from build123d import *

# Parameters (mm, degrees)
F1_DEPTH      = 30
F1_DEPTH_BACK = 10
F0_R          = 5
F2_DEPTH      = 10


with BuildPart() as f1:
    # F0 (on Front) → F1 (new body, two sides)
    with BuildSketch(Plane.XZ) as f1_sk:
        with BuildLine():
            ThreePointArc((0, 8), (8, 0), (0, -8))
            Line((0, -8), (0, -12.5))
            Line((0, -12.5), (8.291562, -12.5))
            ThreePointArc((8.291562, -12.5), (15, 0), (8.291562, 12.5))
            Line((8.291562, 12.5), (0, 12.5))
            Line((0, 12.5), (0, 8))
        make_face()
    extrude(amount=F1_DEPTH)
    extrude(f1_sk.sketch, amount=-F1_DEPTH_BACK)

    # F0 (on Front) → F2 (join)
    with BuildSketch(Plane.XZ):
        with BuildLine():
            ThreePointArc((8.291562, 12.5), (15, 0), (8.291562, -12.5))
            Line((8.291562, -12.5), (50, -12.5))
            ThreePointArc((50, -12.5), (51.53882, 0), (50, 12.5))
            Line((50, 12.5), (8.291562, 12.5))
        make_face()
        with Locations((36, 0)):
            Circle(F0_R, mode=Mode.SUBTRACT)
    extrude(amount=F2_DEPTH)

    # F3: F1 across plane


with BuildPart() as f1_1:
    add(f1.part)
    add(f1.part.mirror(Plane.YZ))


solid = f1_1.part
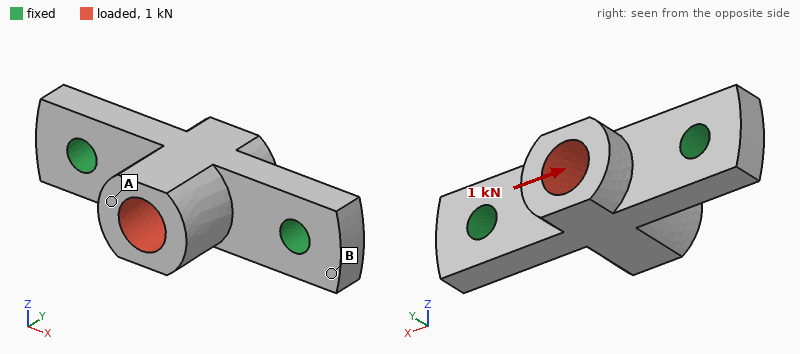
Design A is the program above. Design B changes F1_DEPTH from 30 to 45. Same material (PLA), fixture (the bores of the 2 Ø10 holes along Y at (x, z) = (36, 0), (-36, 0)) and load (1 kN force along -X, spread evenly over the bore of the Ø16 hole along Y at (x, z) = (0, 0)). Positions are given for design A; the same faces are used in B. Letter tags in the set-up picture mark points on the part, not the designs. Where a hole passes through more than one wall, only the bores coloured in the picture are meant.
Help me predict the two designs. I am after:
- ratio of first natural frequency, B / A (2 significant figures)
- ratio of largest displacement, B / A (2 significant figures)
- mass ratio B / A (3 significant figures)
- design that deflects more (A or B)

0.58
2.9
1.19
B
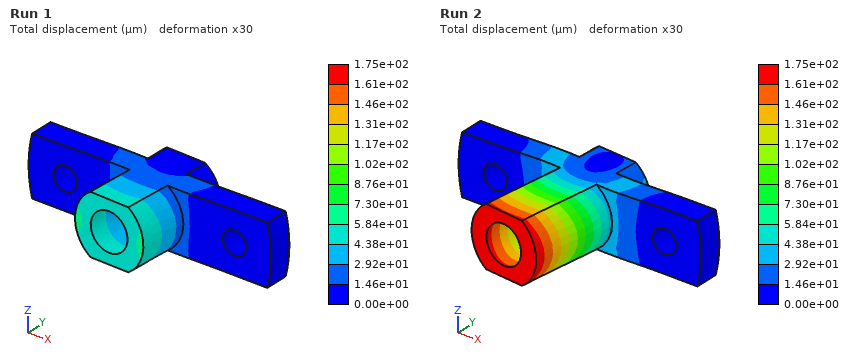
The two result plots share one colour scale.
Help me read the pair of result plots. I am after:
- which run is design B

Run 2
